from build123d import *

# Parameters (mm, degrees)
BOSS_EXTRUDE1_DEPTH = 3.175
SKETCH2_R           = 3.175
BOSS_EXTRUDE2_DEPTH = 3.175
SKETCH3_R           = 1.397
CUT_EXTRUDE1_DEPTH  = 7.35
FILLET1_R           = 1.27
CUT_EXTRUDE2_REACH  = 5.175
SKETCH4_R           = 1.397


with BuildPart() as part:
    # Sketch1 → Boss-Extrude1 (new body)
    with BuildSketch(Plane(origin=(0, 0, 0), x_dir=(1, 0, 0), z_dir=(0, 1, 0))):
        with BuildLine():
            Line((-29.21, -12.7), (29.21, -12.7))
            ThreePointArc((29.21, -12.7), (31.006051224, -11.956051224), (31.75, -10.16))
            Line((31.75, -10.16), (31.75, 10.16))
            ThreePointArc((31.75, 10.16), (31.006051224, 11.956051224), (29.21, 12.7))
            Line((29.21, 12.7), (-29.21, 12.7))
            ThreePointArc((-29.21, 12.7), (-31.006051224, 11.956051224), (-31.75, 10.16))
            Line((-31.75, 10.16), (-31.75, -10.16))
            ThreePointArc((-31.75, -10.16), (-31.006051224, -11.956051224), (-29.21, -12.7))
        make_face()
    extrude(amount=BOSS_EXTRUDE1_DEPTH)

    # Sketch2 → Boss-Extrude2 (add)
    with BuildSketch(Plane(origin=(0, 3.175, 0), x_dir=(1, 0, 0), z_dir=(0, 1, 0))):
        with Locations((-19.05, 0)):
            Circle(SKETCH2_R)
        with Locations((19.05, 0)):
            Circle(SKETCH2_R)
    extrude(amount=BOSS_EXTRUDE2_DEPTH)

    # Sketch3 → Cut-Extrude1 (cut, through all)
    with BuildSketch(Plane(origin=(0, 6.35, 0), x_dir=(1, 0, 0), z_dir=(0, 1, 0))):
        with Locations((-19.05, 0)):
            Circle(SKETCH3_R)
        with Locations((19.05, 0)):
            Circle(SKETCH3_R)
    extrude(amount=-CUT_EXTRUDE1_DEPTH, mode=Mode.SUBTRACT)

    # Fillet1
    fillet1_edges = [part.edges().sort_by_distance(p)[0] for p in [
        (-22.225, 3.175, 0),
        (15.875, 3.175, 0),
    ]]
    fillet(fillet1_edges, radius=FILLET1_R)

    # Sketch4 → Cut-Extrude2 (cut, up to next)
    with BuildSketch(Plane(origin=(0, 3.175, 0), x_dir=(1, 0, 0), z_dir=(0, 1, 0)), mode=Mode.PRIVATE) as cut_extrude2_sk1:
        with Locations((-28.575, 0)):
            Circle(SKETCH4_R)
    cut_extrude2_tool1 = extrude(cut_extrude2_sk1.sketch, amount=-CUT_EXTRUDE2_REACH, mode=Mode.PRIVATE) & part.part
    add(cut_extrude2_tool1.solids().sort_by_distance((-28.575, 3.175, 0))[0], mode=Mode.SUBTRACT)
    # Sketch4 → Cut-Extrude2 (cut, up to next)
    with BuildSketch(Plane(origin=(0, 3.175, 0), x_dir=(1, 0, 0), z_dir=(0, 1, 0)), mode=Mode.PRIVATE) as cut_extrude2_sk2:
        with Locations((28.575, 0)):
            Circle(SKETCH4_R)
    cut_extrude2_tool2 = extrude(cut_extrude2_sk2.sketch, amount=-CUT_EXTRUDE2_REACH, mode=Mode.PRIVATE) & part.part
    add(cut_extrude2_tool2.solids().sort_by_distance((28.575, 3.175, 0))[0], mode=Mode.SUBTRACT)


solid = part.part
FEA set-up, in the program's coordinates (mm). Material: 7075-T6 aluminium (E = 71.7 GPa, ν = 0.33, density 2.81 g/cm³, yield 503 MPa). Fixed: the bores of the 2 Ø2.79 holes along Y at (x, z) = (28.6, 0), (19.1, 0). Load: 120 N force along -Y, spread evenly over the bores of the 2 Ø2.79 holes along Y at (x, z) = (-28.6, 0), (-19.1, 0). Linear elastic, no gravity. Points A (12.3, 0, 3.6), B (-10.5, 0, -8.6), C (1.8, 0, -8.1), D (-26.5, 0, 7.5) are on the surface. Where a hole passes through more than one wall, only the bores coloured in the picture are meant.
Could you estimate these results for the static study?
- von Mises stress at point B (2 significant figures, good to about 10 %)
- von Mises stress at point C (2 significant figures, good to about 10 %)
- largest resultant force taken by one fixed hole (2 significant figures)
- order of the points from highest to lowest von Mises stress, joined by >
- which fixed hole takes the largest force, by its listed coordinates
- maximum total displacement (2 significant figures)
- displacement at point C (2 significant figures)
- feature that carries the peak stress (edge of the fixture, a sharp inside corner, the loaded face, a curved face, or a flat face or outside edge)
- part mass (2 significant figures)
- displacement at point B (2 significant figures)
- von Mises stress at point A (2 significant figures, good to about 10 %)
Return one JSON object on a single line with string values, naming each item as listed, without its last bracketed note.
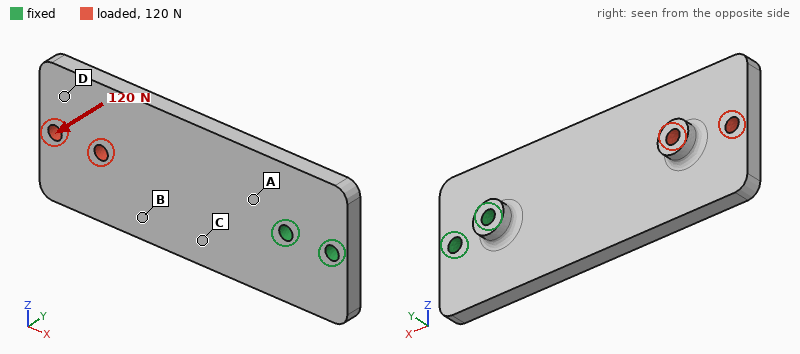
{"von Mises stress at point B": "33 MPa", "von Mises stress at point C": "66 MPa", "largest resultant force taken by one fixed hole": "270 N", "order of the points from highest to lowest von Mises stress, joined by >": "A > C > B > D", "which fixed hole takes the largest force, by its listed coordinates": "(19.1, 0)", "maximum total displacement": "0.75 mm", "displacement at point C": "0.12 mm", "feature that carries the peak stress": "a curved face", "part mass": "15 g", "displacement at point B": "0.32 mm", "von Mises stress at point A": "95 MPa"}
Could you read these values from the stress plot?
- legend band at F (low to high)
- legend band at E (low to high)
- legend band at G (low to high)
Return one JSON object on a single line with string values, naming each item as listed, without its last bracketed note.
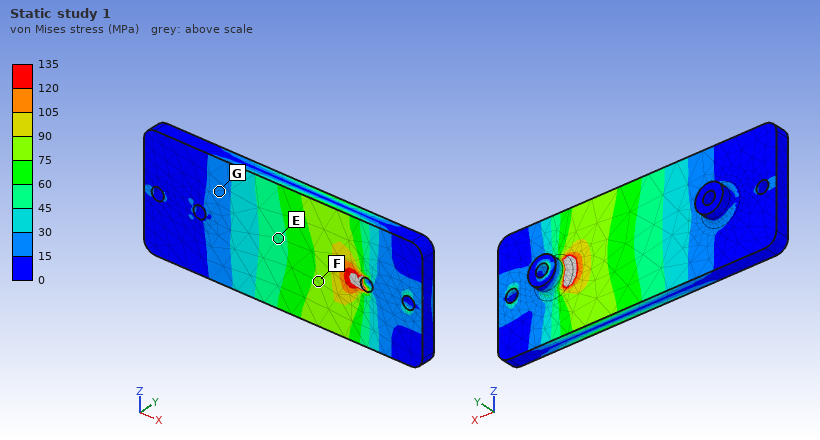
{"legend band at F": "75 to 90 MPa", "legend band at E": "45 to 60 MPa", "legend band at G": "15 to 30 MPa"}
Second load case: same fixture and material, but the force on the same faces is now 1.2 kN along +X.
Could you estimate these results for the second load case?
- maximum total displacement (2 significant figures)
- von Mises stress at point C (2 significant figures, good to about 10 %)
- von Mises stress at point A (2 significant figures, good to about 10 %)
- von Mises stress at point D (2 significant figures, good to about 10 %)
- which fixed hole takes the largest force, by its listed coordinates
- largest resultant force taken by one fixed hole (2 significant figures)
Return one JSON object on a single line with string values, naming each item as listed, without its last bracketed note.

{"maximum total displacement": "0.29 mm", "von Mises stress at point C": "15 MPa", "von Mises stress at point A": "15 MPa", "von Mises stress at point D": "7.9 MPa", "which fixed hole takes the largest force, by its listed coordinates": "(19.1, 0)", "largest resultant force taken by one fixed hole": "950 N"}
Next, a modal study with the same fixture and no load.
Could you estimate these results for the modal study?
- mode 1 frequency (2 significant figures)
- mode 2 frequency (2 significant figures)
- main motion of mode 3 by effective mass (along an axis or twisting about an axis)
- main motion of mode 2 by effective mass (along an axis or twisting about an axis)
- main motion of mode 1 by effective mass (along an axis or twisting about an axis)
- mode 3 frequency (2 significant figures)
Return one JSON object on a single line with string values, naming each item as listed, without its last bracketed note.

{"mode 1 frequency": "1000 Hz", "mode 2 frequency": "3800 Hz", "main motion of mode 3 by effective mass": "along Z", "main motion of mode 2 by effective mass": "twisting about X", "main motion of mode 1 by effective mass": "along Y", "mode 3 frequency": "4500 Hz"}
